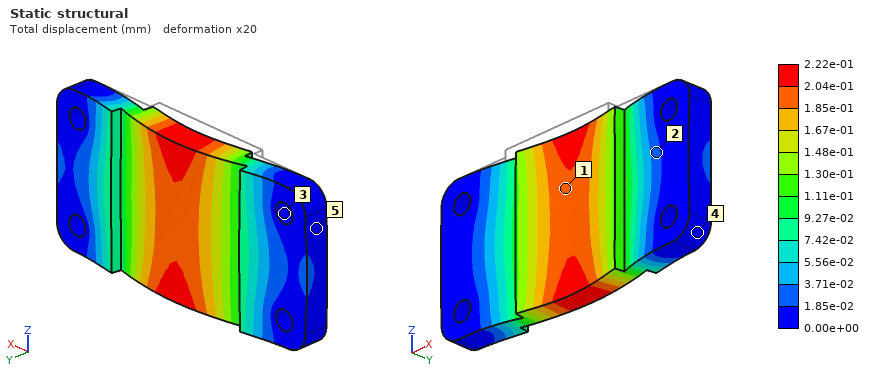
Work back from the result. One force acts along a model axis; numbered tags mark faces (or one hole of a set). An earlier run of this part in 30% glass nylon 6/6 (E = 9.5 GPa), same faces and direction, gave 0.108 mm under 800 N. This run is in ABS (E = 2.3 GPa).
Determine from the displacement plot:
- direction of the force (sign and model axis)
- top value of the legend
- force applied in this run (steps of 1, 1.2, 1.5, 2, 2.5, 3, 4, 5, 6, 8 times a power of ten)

+Y
2.22e-01 mm
400 N
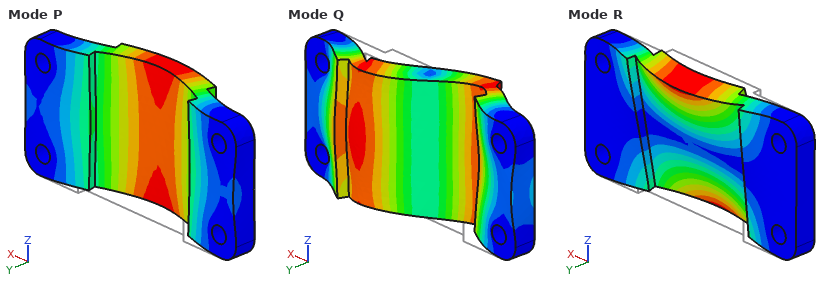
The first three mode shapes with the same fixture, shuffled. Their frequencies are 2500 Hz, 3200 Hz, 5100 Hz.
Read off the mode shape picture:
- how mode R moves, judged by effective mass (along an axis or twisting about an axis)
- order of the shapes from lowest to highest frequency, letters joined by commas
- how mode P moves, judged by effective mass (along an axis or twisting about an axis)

twisting about X
P, R, Q
along Y
